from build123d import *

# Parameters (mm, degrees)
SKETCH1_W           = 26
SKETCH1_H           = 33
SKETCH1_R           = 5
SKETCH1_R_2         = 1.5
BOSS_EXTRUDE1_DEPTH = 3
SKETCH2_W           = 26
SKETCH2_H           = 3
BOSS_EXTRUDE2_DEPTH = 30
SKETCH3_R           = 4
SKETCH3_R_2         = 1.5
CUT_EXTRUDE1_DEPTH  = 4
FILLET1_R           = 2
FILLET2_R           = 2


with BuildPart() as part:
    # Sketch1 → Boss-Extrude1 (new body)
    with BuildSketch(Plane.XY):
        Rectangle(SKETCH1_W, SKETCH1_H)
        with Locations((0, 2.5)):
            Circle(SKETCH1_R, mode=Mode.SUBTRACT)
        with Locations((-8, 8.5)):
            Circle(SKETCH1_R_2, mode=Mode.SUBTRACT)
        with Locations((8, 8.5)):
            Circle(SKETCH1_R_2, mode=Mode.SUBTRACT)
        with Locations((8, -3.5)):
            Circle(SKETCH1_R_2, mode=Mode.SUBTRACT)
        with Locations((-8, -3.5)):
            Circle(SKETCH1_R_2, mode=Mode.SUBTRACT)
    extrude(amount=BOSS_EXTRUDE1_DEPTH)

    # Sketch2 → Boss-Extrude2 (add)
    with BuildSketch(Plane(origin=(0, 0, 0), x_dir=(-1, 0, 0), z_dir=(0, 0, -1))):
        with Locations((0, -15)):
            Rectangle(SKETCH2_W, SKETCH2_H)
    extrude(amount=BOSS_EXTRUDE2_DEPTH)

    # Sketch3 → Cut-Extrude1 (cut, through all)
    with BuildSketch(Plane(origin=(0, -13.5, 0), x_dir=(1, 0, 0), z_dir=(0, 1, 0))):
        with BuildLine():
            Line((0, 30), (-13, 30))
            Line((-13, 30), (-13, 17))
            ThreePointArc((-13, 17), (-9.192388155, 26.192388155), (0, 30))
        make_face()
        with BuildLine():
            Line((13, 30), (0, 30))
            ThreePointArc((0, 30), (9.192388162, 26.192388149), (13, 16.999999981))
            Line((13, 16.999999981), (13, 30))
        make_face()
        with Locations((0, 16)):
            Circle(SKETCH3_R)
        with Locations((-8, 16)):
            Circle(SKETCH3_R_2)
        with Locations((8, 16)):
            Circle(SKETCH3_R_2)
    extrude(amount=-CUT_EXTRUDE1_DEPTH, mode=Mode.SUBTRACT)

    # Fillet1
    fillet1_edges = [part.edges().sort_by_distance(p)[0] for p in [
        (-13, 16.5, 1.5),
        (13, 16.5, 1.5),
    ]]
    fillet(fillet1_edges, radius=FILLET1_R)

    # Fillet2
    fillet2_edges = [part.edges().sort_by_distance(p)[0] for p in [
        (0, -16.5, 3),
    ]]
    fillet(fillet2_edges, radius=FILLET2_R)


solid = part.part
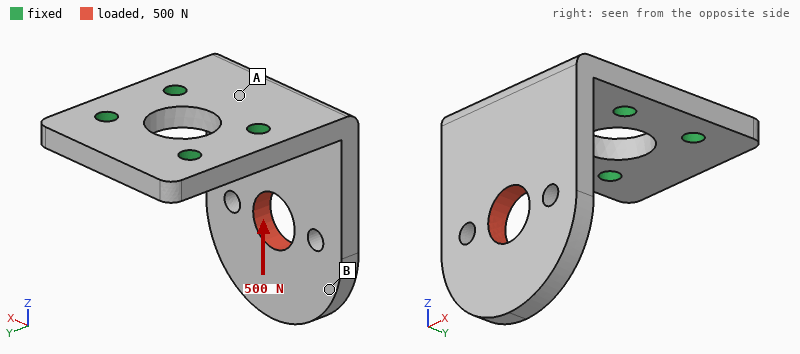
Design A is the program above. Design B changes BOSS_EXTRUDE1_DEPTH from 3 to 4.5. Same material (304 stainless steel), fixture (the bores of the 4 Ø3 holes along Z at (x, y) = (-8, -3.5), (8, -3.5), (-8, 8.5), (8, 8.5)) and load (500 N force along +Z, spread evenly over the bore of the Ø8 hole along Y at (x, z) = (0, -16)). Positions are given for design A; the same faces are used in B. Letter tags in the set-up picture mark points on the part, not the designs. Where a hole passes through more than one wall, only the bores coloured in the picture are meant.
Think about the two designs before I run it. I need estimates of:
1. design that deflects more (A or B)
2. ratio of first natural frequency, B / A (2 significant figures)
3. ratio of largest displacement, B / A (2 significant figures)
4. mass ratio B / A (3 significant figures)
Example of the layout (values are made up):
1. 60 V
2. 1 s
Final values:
1. A
2. 1.3
3. 0.34
4. 1.27
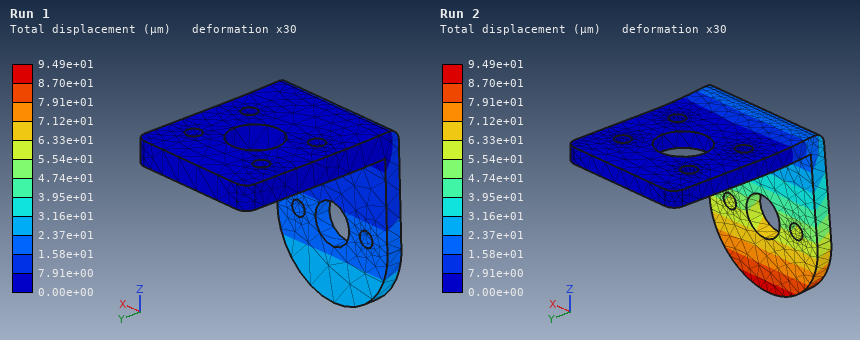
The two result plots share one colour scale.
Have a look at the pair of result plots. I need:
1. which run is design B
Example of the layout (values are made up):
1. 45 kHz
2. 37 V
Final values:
1. Run 1
